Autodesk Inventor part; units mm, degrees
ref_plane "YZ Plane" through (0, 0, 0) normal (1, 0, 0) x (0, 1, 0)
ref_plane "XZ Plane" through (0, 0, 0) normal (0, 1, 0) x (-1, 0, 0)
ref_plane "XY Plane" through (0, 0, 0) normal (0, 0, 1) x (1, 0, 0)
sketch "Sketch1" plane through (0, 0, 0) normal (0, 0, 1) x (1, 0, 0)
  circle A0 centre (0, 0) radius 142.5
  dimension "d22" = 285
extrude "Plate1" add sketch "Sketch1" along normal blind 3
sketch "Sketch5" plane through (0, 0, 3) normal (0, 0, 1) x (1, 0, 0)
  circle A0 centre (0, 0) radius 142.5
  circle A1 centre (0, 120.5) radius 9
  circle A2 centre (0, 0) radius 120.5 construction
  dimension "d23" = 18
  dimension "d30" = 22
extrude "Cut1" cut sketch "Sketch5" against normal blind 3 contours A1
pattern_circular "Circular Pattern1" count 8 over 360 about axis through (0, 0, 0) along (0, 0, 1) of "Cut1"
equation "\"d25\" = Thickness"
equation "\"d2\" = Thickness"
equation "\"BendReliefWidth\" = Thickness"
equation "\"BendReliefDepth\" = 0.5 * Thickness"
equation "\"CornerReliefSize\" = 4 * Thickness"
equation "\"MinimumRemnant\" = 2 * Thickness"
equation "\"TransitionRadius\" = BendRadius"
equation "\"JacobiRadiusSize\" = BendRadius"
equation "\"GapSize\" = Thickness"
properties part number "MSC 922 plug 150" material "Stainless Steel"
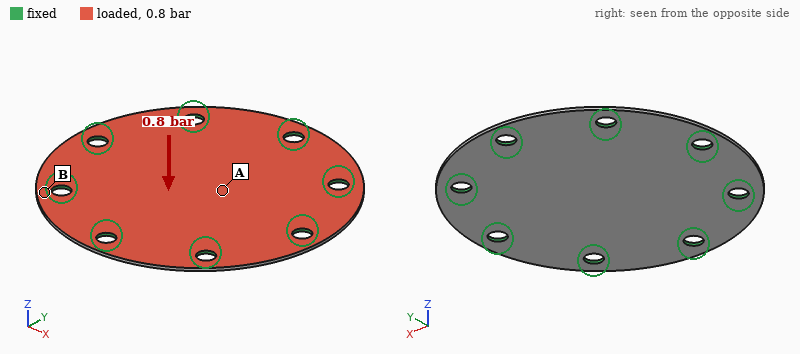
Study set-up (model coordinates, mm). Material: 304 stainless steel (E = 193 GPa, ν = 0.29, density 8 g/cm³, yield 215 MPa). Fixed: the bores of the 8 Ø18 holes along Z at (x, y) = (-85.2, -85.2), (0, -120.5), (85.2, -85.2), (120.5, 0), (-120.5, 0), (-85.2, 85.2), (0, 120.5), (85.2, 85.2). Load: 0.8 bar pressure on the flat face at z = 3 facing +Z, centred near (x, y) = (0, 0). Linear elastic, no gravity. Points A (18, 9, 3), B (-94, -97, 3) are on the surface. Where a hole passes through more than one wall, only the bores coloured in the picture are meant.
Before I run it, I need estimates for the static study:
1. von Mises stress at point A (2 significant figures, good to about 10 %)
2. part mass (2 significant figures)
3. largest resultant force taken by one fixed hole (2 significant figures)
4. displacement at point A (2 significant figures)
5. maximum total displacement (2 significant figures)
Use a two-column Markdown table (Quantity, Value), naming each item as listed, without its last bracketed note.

| Quantity | Value |
|---|---|
| von Mises stress at point A | 56 MPa |
| part mass | 1.5 kg |
| largest resultant force taken by one fixed hole | 620 N |
| displacement at point A | 0.49 mm |
| maximum total displacement | 0.52 mm |
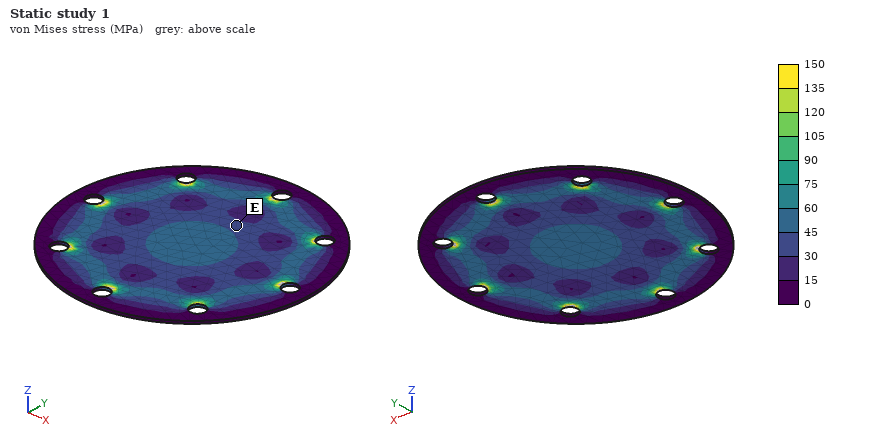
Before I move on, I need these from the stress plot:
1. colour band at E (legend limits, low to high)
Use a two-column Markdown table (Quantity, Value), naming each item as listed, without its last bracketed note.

| Quantity | Value |
|---|---|
| colour band at E | 30 to 45 MPa |
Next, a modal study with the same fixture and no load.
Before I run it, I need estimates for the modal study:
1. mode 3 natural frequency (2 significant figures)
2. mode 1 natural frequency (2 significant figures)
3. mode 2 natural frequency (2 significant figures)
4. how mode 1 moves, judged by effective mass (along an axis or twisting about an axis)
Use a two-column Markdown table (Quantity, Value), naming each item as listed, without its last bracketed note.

| Quantity | Value |
|---|---|
| mode 3 natural frequency | 1000 Hz |
| mode 1 natural frequency | 510 Hz |
| mode 2 natural frequency | 1000 Hz |
| how mode 1 moves, judged by effective mass | along Z |
